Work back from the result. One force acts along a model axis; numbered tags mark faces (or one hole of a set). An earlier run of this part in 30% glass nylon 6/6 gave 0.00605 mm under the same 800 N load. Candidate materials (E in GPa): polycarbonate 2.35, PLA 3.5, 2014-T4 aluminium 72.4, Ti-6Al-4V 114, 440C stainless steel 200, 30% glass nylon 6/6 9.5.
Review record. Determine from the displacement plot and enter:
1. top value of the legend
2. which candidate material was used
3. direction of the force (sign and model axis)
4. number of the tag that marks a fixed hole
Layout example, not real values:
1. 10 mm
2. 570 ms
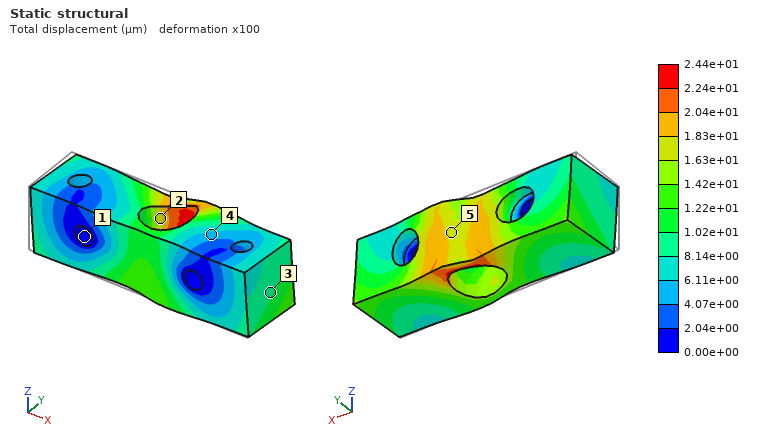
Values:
1. 2.44e+01 µm
2. polycarbonate
3. +X
4. 1
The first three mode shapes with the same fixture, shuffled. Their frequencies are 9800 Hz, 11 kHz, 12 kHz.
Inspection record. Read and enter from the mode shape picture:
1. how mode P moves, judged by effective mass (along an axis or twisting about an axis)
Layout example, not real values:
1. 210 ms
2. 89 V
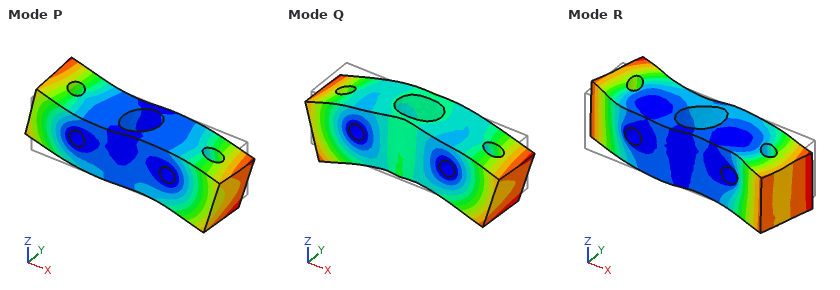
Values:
1. twisting about Y
